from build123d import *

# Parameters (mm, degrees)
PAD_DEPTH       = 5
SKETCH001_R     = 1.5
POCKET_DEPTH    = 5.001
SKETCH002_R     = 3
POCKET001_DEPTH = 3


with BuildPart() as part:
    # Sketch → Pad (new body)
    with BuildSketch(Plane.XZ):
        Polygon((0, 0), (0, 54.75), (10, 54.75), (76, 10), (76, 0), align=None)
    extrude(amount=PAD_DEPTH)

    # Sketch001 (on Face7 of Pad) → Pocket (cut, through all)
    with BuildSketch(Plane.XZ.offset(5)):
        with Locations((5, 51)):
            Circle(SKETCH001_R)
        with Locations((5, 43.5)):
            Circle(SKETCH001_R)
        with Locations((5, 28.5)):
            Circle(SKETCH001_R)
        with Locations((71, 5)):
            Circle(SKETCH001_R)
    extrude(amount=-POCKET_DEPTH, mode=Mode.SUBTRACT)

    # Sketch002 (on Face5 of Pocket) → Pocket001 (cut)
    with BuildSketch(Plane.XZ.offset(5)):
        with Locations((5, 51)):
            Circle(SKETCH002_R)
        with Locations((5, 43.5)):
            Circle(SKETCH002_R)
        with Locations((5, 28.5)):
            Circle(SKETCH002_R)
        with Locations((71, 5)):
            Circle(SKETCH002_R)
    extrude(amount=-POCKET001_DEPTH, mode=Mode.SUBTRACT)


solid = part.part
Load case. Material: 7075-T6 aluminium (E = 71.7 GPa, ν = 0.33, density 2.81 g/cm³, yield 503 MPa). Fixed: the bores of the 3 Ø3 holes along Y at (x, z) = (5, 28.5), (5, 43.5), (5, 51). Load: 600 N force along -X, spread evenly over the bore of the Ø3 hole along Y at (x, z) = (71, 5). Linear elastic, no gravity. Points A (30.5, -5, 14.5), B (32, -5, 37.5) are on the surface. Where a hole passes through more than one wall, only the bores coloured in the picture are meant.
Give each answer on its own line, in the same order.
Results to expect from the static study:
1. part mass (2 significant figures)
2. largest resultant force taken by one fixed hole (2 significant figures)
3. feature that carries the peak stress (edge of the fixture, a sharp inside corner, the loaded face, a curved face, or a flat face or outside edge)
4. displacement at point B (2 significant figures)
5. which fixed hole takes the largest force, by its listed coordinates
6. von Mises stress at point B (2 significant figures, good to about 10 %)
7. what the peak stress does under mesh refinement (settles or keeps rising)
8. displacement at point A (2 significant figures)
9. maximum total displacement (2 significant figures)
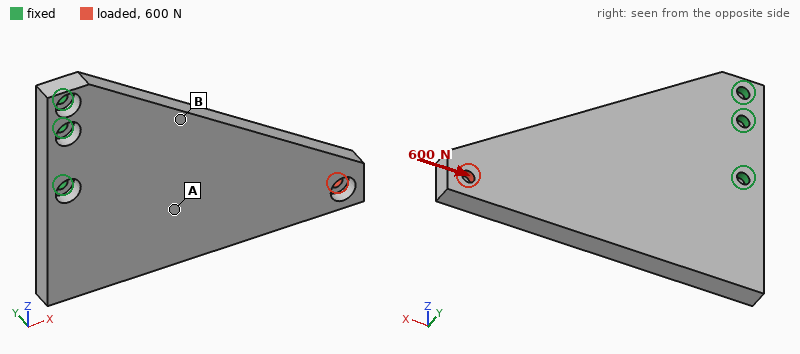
37 g
1.2 kN
edge of the fixture
14 µm
(5, 28.5)
12 MPa
keeps rising
20 µm
91 µm
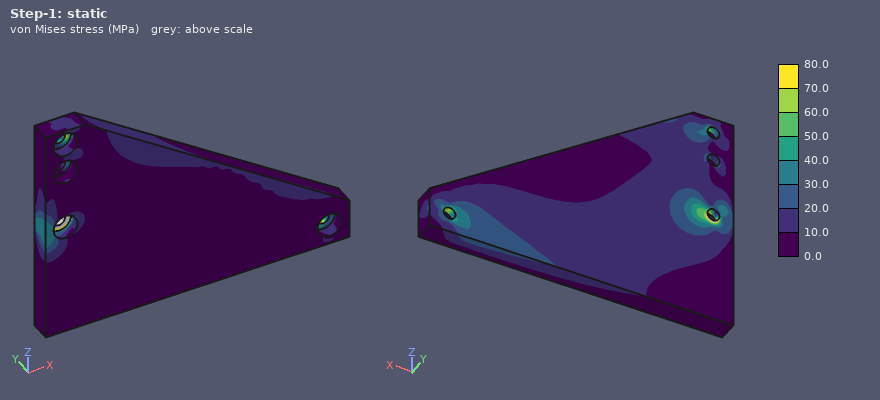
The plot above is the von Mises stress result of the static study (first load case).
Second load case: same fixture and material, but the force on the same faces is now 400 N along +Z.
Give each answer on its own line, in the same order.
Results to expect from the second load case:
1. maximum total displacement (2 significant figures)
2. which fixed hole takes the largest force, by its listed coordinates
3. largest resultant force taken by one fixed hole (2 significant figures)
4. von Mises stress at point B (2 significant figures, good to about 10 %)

0.13 mm
(5, 28.5)
1.2 kN
15 MPa
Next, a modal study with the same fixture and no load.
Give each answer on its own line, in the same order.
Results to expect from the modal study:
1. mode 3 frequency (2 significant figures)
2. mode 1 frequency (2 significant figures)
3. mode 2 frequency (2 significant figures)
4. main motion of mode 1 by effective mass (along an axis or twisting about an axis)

3900 Hz
740 Hz
3100 Hz
along Y
